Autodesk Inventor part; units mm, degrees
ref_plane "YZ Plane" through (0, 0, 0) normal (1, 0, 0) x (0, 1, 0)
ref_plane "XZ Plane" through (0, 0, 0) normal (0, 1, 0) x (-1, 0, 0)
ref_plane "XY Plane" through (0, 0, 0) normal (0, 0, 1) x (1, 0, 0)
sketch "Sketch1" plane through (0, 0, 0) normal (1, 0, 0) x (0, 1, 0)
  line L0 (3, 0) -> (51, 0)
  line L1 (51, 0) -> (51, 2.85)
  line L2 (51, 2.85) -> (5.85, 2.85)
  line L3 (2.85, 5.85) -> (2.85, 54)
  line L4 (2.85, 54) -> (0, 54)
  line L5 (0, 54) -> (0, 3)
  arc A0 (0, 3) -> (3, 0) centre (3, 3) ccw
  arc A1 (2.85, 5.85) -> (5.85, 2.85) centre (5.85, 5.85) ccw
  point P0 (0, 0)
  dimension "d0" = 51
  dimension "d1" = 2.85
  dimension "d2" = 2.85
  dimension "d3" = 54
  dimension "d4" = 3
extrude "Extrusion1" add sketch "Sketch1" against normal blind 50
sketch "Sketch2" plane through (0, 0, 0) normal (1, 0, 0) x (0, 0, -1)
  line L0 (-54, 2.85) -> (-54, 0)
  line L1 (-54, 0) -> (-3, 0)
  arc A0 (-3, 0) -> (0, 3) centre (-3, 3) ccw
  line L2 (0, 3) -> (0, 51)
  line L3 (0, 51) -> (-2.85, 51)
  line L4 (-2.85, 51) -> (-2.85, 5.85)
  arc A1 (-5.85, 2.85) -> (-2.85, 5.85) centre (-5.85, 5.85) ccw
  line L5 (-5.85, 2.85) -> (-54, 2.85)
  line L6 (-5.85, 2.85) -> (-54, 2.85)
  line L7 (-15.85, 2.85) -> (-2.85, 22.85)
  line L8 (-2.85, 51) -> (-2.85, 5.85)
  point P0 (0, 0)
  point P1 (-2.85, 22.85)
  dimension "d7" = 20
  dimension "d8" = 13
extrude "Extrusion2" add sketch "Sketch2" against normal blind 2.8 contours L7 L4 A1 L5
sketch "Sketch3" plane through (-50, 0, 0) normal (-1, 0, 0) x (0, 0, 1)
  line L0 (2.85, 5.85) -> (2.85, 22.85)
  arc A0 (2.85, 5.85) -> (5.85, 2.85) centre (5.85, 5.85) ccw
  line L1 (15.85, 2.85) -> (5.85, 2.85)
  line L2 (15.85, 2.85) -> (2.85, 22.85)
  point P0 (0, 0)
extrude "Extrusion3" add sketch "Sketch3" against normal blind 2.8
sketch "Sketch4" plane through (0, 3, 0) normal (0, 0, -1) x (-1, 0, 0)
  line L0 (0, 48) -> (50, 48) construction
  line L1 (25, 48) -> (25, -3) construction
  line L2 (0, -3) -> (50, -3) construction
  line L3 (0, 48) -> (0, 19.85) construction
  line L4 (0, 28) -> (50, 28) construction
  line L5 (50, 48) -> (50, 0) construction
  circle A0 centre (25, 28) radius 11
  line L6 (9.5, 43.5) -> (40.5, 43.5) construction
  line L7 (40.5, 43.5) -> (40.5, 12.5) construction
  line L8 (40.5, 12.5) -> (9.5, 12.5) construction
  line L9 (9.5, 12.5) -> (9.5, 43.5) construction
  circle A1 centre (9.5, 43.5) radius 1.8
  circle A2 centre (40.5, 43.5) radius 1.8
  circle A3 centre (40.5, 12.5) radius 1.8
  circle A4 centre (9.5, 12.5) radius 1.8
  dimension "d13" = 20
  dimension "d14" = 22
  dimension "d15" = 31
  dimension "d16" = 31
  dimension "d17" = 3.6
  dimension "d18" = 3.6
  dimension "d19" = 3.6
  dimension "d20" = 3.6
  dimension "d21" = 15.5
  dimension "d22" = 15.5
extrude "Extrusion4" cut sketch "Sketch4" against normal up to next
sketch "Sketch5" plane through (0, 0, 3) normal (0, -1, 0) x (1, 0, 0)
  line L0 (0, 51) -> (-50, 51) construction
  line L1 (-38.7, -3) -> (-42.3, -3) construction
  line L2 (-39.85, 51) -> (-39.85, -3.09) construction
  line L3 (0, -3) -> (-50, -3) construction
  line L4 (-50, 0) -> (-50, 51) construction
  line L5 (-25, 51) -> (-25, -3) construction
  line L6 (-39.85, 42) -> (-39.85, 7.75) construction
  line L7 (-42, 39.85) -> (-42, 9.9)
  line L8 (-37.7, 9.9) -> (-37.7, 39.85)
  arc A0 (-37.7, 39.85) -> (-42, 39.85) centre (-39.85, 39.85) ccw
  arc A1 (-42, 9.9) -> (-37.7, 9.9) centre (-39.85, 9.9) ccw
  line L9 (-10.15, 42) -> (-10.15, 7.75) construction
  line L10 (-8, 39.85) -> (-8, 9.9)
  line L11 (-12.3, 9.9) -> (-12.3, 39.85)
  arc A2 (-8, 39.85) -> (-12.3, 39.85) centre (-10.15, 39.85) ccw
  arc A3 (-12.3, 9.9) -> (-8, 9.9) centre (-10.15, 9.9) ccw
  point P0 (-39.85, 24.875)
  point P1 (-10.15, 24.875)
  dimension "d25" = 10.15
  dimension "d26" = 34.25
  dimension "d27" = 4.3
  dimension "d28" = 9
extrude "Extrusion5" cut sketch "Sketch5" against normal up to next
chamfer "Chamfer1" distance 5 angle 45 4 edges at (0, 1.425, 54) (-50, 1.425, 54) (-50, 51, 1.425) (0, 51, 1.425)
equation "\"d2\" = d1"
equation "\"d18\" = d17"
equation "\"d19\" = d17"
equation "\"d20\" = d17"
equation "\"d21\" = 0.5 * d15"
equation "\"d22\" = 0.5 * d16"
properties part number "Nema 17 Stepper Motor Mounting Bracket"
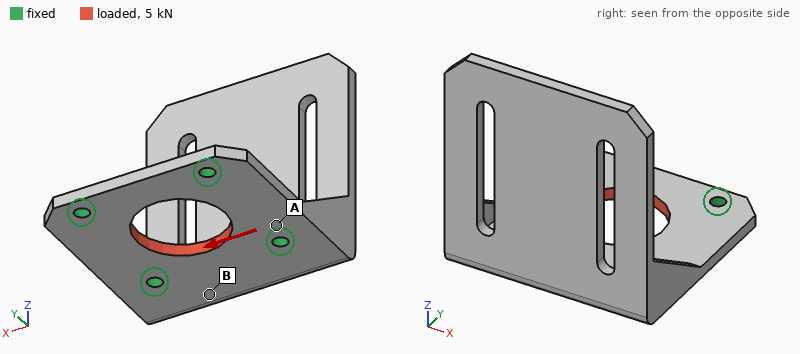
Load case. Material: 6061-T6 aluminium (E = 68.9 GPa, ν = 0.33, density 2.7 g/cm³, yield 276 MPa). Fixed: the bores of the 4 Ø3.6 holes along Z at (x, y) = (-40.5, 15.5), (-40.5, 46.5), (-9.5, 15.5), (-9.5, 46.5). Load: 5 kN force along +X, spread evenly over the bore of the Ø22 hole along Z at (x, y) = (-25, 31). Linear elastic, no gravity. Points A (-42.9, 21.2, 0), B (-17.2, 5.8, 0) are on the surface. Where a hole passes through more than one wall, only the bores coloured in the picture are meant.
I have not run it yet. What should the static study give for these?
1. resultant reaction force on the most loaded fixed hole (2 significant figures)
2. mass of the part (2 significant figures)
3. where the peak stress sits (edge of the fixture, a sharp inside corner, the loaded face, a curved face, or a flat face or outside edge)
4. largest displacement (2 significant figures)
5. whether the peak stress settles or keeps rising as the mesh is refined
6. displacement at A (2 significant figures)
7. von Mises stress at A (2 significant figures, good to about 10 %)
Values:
1.3 kN
35 g
edge of the fixture
12 µm
keeps rising
5.0 µm
29 MPa
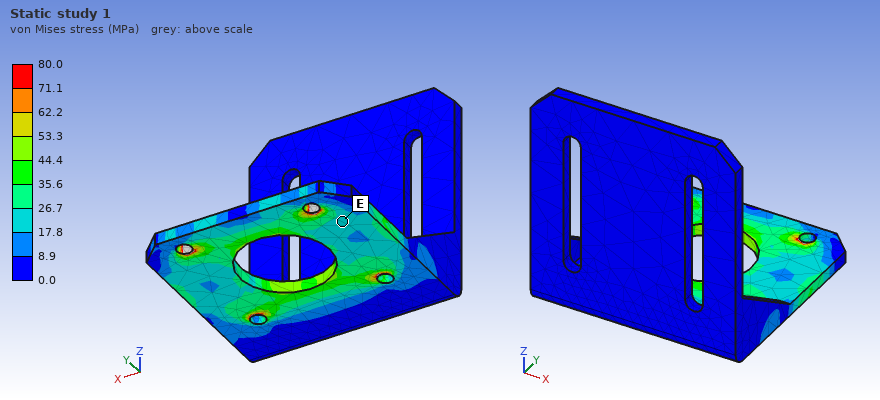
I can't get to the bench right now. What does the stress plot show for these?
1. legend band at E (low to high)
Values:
17.8 to 26.7 MPa
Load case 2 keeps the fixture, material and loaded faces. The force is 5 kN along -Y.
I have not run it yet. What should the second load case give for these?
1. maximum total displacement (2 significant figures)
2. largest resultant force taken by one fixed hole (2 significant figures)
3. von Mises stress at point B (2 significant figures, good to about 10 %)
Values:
17 µm
1.3 kN
15 MPa
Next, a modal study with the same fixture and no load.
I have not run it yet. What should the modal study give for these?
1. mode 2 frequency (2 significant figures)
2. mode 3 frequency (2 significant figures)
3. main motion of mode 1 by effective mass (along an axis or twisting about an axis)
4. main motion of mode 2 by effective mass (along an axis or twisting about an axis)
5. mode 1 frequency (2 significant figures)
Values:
2000 Hz
3000 Hz
along Y
along X
870 Hz
